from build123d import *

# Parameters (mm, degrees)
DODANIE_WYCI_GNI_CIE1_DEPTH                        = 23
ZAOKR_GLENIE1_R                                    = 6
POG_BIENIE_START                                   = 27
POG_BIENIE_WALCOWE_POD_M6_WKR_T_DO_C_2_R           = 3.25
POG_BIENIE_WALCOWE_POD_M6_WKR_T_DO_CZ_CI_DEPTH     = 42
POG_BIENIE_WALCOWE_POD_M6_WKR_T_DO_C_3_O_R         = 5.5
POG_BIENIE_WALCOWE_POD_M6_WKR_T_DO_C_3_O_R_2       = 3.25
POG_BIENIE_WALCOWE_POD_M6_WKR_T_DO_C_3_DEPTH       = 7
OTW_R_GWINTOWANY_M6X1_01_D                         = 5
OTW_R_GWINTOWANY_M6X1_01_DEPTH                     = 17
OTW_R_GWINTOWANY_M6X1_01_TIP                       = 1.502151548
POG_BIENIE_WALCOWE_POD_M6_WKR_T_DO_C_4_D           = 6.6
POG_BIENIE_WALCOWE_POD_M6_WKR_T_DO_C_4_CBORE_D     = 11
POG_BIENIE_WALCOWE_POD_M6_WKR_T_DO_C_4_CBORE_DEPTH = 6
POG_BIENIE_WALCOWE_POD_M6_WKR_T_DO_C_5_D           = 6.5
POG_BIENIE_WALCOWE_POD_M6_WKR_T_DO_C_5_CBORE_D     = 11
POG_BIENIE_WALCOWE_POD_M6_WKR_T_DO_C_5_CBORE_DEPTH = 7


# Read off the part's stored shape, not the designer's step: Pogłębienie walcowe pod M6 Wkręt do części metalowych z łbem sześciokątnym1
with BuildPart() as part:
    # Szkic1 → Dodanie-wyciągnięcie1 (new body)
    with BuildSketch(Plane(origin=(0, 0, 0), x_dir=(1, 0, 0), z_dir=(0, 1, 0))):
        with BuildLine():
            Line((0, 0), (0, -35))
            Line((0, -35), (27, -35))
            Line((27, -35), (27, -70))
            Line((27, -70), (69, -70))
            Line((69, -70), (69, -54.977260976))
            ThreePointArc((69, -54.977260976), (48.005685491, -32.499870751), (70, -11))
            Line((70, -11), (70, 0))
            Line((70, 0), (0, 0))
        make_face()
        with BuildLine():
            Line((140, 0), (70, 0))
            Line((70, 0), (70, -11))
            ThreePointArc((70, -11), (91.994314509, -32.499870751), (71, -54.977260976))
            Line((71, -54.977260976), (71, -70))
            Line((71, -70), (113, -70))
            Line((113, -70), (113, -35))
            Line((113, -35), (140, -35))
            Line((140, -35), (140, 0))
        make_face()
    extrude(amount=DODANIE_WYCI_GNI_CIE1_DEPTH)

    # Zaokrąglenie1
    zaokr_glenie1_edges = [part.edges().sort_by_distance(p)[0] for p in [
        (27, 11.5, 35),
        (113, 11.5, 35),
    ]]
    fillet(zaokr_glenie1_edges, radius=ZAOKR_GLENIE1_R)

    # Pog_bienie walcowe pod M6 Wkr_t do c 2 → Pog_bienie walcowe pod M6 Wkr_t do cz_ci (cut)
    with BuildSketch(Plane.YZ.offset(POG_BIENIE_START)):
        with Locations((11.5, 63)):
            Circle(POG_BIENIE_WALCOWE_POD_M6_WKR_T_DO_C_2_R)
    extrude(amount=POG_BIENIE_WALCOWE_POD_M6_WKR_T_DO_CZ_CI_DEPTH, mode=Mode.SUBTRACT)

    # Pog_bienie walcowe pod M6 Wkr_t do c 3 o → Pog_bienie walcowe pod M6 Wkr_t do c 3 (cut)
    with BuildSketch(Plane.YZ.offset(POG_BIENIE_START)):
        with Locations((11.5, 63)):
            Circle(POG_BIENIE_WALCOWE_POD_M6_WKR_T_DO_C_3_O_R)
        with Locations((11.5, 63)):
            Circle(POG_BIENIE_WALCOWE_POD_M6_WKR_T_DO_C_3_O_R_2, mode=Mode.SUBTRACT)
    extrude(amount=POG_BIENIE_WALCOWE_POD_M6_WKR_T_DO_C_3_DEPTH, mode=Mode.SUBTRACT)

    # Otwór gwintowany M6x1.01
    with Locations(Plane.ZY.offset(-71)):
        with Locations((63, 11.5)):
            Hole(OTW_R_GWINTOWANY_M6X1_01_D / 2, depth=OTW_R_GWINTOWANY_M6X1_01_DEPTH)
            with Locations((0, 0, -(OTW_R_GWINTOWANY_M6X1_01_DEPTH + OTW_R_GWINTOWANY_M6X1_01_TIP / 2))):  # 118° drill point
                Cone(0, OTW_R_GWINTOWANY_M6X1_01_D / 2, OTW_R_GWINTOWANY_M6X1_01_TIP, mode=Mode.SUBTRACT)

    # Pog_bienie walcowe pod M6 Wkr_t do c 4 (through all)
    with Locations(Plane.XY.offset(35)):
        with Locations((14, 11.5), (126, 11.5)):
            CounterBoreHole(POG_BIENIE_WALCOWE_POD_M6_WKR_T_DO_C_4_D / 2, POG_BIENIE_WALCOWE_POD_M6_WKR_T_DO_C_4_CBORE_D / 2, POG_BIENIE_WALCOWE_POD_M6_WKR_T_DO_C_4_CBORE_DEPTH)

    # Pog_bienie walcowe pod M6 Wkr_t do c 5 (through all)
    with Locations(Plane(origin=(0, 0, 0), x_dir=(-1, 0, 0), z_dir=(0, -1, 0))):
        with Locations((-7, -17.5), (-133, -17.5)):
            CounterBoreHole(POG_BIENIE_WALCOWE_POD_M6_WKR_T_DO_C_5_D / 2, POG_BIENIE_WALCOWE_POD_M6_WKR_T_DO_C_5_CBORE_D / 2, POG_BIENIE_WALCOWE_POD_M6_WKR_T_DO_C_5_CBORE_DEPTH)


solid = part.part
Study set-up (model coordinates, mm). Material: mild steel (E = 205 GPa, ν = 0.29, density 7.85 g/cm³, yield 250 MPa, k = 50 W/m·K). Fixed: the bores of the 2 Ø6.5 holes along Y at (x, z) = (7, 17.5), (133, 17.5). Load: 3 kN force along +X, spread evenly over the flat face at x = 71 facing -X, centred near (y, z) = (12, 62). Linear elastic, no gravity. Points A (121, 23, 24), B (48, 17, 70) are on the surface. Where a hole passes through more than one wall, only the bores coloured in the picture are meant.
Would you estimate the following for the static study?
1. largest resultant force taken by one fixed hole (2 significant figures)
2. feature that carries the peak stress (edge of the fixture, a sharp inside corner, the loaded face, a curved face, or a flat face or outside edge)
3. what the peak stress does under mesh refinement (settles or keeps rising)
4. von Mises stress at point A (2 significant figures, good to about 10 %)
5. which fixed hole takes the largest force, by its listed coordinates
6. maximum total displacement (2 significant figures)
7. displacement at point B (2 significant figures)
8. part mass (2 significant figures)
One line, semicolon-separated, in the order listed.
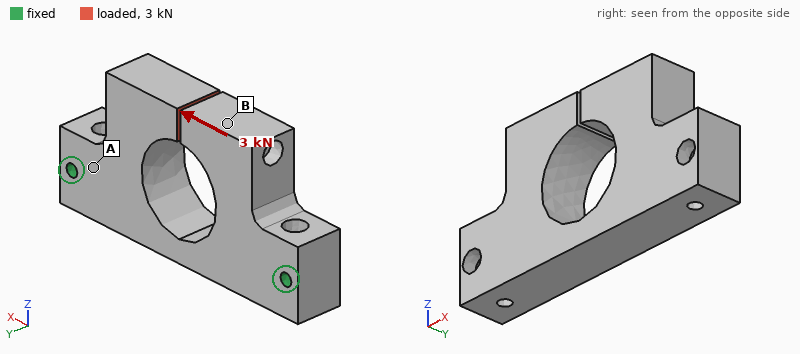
5.4 kN; edge of the fixture; keeps rising; 14 MPa; (133, 17.5); 51 µm; 14 µm; 1.1 kg
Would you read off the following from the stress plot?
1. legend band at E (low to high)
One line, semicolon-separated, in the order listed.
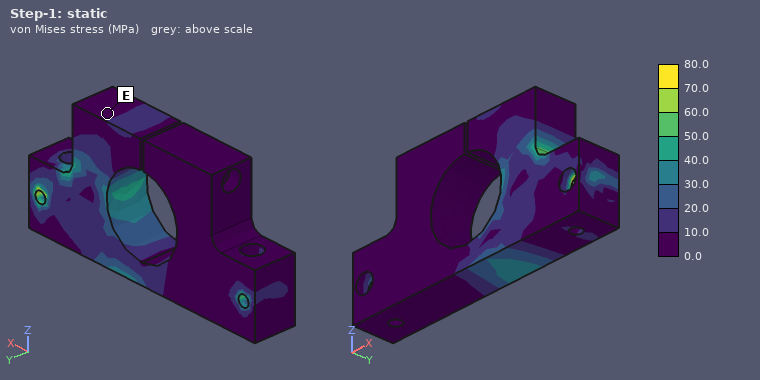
0.0 to 10.0 MPa
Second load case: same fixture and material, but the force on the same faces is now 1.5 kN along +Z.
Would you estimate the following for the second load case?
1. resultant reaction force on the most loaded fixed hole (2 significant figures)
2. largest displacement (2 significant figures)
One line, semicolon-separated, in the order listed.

2.0 kN; 34 µm
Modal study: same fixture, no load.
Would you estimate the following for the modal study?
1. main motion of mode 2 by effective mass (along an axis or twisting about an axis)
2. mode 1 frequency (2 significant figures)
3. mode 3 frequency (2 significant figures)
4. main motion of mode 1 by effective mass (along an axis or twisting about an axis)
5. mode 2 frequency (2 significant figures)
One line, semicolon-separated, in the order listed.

along Z; 2300 Hz; 2700 Hz; along Y; 2600 Hz
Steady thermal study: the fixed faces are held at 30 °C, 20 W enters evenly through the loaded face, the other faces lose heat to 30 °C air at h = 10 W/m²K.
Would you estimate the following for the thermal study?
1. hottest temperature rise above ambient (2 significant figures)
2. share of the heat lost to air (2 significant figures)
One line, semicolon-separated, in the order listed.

59 K; 15 %
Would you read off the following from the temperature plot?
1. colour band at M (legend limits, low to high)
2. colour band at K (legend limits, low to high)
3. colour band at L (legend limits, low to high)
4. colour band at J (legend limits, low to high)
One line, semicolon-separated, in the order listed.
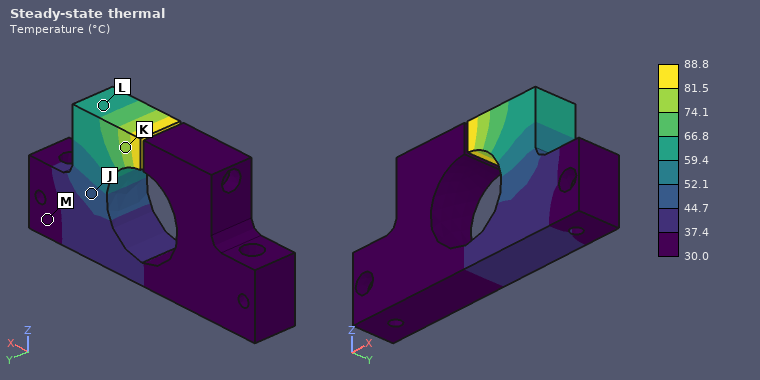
30.0 to 37.4 °C; 74.1 to 81.5 °C; 59.4 to 66.8 °C; 44.7 to 52.1 °C
